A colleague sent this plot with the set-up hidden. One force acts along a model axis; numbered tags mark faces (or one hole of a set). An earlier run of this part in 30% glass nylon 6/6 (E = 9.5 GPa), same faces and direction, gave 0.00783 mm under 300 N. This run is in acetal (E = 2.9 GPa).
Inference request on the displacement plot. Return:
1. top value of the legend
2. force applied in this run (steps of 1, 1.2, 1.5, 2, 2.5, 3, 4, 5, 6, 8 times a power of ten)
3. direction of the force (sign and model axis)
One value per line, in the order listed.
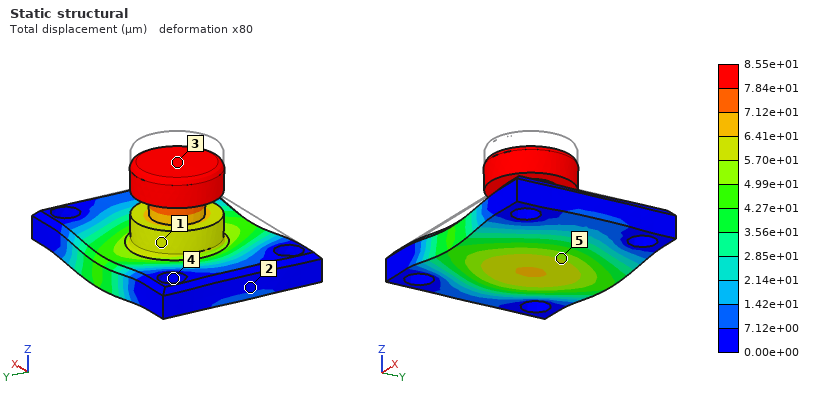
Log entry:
8.55e+01 µm
1 kN
-Z
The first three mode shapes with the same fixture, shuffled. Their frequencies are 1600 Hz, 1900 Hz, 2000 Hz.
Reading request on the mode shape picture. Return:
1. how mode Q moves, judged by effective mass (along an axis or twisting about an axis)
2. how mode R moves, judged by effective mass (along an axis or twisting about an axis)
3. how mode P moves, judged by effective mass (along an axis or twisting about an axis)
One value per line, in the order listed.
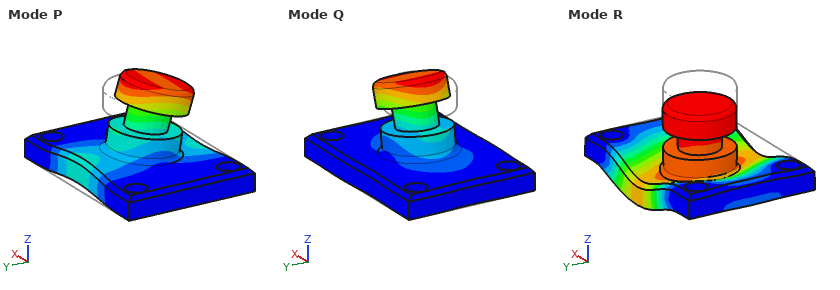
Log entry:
along X
along Z
along Y
